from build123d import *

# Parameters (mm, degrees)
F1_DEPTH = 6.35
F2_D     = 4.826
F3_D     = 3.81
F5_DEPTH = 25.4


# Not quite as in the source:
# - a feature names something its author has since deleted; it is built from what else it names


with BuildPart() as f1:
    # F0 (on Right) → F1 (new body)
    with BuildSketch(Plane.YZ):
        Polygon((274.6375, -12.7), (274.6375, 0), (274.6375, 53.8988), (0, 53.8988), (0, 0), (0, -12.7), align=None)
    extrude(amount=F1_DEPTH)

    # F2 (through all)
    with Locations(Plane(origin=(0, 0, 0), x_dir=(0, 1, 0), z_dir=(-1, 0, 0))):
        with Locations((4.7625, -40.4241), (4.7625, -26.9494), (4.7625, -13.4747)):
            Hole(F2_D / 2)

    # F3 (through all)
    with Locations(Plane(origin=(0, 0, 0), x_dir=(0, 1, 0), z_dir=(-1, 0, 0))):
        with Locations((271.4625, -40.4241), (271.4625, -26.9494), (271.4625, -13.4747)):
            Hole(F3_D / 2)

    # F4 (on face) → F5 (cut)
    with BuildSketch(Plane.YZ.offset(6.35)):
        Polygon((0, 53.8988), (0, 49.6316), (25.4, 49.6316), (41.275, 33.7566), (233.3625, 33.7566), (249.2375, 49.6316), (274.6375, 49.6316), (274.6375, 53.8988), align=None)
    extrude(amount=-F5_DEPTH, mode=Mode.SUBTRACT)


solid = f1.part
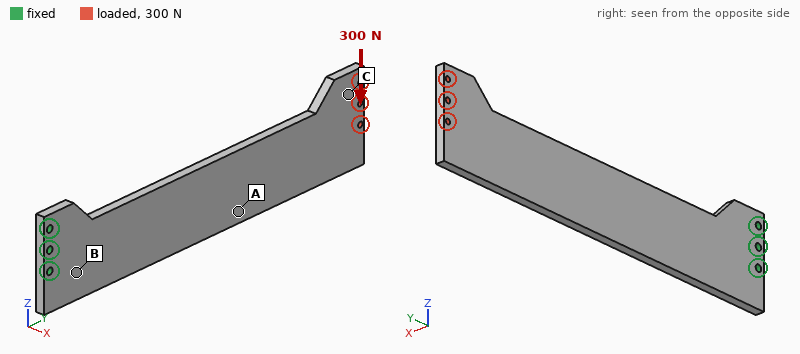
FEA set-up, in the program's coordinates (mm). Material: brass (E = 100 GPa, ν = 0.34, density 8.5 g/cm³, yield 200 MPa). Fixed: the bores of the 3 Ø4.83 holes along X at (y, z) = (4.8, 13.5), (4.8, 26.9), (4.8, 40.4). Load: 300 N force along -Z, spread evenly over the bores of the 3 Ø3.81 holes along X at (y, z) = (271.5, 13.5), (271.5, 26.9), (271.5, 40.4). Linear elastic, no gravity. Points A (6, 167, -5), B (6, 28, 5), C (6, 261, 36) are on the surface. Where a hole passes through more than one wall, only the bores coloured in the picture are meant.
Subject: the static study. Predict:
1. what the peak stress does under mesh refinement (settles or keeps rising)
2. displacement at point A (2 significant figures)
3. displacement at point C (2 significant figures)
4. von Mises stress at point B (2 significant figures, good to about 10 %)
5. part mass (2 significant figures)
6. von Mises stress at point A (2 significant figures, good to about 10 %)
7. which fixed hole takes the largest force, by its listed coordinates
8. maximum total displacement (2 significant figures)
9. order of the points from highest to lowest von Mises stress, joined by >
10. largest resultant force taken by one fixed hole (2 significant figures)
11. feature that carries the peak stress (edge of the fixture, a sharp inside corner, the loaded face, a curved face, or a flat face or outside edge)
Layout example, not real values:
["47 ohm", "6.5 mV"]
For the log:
["keeps rising", "0.18 mm", "0.38 mm", "16 MPa", "740 g", "9.3 MPa", "(4.8, 13.5)", "0.41 mm", "B > A > C", "2.8 kN", "edge of the fixture"]
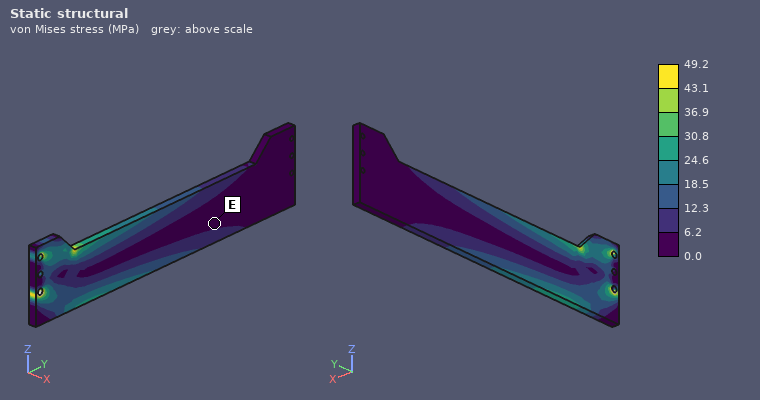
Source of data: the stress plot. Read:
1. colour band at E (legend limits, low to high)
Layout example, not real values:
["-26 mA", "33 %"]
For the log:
["0.0 to 6.2 MPa"]
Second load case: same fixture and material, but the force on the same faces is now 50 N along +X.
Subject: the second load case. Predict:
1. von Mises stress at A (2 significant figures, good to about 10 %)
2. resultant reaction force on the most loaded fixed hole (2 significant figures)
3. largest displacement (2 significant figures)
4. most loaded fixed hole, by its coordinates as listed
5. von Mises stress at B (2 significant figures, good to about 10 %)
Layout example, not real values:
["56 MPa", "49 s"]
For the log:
["17 MPa", "130 N", "3.1 mm", "(4.8, 26.9)", "31 MPa"]
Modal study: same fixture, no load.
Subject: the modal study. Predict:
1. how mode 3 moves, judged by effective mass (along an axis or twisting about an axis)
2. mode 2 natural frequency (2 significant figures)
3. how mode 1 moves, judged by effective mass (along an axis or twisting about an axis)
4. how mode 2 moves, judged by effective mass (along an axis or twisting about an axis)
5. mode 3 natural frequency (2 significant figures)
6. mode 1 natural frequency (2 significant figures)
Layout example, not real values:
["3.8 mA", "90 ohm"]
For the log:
["along Z", "290 Hz", "along X", "along X", "310 Hz", "47 Hz"]
